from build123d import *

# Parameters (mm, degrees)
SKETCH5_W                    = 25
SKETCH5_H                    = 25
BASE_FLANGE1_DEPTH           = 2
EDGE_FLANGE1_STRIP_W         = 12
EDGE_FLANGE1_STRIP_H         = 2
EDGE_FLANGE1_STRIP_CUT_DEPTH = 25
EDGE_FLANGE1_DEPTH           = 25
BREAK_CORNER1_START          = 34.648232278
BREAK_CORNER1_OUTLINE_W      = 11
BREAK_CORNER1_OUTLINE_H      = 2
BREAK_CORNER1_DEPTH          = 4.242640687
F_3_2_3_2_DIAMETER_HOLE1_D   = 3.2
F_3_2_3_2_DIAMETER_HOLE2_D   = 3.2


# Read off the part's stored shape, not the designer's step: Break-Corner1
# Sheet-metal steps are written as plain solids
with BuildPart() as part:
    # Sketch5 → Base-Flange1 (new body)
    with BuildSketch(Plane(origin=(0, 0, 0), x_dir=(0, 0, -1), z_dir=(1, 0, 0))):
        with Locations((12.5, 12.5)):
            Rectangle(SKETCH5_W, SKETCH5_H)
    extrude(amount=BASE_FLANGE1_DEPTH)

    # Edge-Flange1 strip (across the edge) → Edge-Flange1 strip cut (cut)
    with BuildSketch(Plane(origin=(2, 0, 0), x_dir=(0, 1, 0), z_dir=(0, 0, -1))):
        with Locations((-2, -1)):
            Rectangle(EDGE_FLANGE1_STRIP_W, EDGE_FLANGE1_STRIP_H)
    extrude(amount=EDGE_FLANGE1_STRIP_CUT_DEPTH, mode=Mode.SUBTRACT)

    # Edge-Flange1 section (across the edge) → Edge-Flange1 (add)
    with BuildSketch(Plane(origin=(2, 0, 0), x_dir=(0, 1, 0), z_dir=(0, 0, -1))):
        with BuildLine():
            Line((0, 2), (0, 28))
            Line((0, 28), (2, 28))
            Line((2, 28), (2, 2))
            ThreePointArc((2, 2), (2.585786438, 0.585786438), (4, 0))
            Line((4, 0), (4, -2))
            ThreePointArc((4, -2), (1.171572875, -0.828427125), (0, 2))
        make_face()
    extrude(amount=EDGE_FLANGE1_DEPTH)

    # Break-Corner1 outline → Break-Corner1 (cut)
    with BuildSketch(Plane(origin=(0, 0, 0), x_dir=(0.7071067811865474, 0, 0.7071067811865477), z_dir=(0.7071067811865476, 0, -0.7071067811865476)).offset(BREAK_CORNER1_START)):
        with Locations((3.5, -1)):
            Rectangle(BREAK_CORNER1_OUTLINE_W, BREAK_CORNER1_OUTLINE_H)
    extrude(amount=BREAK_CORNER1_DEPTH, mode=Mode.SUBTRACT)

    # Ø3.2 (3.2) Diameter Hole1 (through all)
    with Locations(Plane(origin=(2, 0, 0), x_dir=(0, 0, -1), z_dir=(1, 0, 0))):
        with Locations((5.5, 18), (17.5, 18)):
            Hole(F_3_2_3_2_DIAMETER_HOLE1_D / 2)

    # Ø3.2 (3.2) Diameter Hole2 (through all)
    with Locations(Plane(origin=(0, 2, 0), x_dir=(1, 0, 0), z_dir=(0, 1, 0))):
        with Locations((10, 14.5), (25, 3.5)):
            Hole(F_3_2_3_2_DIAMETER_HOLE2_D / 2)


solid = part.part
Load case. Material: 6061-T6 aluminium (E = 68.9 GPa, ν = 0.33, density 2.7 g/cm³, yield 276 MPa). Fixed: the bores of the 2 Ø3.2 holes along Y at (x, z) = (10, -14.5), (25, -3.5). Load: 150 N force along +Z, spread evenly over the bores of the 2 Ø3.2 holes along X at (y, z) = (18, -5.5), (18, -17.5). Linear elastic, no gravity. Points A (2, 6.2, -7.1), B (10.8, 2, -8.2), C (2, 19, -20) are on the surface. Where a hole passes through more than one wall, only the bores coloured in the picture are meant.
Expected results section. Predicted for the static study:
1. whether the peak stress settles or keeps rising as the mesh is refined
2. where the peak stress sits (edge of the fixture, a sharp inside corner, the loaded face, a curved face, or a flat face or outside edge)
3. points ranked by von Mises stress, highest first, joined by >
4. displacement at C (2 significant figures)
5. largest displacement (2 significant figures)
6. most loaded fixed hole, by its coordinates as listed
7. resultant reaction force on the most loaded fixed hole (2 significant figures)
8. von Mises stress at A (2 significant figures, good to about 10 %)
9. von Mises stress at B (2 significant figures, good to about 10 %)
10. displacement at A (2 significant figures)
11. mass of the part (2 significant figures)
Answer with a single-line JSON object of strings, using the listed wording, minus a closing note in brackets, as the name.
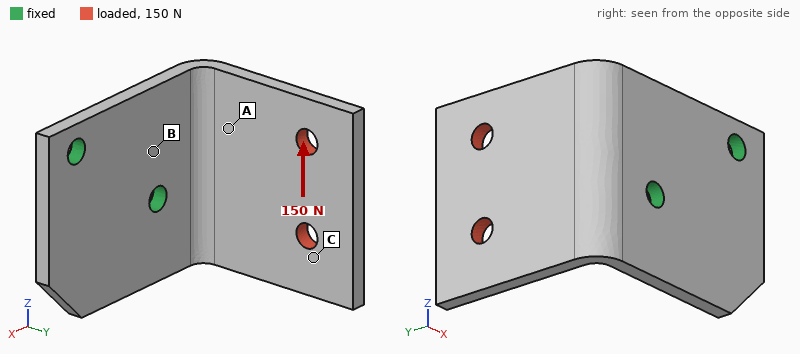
{"whether the peak stress settles or keeps rising as the mesh is refined": "keeps rising", "where the peak stress sits": "edge of the fixture", "points ranked by von Mises stress, highest first, joined by >": "B > A > C", "displacement at C": "0.21 mm", "largest displacement": "0.32 mm", "most loaded fixed hole, by its coordinates as listed": "(10, -14.5)", "resultant reaction force on the most loaded fixed hole": "190 N", "von Mises stress at A": "41 MPa", "von Mises stress at B": "74 MPa", "displacement at A": "0.098 mm", "mass of the part": "6.7 g"}
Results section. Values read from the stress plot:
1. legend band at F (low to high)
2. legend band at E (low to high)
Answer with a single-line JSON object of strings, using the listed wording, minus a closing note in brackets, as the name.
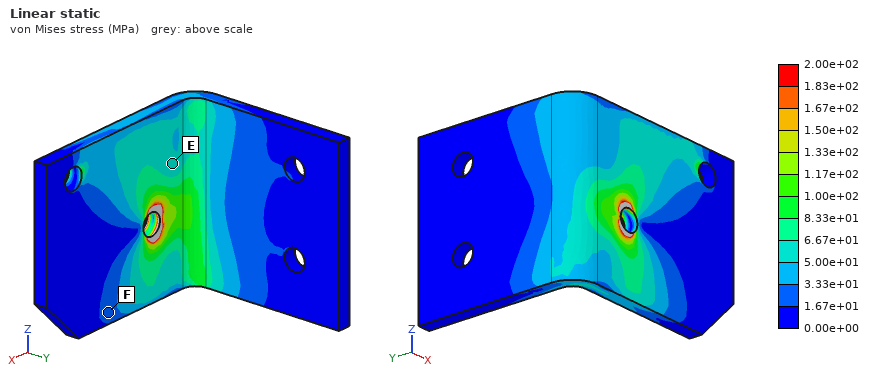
{"legend band at F": "1.67e+01 to 3.33e+01 MPa", "legend band at E": "5.00e+01 to 6.67e+01 MPa"}
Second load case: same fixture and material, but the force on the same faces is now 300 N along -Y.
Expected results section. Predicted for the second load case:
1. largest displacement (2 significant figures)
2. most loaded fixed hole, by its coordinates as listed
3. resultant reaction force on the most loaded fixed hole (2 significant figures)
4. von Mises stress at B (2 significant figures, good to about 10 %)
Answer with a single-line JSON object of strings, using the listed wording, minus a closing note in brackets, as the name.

{"largest displacement": "0.34 mm", "most loaded fixed hole, by its coordinates as listed": "(10, -14.5)", "resultant reaction force on the most loaded fixed hole": "330 N", "von Mises stress at B": "78 MPa"}
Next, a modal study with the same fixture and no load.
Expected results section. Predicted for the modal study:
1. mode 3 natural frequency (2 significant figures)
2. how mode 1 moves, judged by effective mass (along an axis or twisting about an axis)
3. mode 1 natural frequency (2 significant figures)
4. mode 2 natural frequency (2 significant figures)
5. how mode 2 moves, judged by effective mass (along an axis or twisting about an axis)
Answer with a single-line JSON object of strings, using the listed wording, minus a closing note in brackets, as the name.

{"mode 3 natural frequency": "6000 Hz", "how mode 1 moves, judged by effective mass": "along X", "mode 1 natural frequency": "1900 Hz", "mode 2 natural frequency": "2700 Hz", "how mode 2 moves, judged by effective mass": "along Z"}
